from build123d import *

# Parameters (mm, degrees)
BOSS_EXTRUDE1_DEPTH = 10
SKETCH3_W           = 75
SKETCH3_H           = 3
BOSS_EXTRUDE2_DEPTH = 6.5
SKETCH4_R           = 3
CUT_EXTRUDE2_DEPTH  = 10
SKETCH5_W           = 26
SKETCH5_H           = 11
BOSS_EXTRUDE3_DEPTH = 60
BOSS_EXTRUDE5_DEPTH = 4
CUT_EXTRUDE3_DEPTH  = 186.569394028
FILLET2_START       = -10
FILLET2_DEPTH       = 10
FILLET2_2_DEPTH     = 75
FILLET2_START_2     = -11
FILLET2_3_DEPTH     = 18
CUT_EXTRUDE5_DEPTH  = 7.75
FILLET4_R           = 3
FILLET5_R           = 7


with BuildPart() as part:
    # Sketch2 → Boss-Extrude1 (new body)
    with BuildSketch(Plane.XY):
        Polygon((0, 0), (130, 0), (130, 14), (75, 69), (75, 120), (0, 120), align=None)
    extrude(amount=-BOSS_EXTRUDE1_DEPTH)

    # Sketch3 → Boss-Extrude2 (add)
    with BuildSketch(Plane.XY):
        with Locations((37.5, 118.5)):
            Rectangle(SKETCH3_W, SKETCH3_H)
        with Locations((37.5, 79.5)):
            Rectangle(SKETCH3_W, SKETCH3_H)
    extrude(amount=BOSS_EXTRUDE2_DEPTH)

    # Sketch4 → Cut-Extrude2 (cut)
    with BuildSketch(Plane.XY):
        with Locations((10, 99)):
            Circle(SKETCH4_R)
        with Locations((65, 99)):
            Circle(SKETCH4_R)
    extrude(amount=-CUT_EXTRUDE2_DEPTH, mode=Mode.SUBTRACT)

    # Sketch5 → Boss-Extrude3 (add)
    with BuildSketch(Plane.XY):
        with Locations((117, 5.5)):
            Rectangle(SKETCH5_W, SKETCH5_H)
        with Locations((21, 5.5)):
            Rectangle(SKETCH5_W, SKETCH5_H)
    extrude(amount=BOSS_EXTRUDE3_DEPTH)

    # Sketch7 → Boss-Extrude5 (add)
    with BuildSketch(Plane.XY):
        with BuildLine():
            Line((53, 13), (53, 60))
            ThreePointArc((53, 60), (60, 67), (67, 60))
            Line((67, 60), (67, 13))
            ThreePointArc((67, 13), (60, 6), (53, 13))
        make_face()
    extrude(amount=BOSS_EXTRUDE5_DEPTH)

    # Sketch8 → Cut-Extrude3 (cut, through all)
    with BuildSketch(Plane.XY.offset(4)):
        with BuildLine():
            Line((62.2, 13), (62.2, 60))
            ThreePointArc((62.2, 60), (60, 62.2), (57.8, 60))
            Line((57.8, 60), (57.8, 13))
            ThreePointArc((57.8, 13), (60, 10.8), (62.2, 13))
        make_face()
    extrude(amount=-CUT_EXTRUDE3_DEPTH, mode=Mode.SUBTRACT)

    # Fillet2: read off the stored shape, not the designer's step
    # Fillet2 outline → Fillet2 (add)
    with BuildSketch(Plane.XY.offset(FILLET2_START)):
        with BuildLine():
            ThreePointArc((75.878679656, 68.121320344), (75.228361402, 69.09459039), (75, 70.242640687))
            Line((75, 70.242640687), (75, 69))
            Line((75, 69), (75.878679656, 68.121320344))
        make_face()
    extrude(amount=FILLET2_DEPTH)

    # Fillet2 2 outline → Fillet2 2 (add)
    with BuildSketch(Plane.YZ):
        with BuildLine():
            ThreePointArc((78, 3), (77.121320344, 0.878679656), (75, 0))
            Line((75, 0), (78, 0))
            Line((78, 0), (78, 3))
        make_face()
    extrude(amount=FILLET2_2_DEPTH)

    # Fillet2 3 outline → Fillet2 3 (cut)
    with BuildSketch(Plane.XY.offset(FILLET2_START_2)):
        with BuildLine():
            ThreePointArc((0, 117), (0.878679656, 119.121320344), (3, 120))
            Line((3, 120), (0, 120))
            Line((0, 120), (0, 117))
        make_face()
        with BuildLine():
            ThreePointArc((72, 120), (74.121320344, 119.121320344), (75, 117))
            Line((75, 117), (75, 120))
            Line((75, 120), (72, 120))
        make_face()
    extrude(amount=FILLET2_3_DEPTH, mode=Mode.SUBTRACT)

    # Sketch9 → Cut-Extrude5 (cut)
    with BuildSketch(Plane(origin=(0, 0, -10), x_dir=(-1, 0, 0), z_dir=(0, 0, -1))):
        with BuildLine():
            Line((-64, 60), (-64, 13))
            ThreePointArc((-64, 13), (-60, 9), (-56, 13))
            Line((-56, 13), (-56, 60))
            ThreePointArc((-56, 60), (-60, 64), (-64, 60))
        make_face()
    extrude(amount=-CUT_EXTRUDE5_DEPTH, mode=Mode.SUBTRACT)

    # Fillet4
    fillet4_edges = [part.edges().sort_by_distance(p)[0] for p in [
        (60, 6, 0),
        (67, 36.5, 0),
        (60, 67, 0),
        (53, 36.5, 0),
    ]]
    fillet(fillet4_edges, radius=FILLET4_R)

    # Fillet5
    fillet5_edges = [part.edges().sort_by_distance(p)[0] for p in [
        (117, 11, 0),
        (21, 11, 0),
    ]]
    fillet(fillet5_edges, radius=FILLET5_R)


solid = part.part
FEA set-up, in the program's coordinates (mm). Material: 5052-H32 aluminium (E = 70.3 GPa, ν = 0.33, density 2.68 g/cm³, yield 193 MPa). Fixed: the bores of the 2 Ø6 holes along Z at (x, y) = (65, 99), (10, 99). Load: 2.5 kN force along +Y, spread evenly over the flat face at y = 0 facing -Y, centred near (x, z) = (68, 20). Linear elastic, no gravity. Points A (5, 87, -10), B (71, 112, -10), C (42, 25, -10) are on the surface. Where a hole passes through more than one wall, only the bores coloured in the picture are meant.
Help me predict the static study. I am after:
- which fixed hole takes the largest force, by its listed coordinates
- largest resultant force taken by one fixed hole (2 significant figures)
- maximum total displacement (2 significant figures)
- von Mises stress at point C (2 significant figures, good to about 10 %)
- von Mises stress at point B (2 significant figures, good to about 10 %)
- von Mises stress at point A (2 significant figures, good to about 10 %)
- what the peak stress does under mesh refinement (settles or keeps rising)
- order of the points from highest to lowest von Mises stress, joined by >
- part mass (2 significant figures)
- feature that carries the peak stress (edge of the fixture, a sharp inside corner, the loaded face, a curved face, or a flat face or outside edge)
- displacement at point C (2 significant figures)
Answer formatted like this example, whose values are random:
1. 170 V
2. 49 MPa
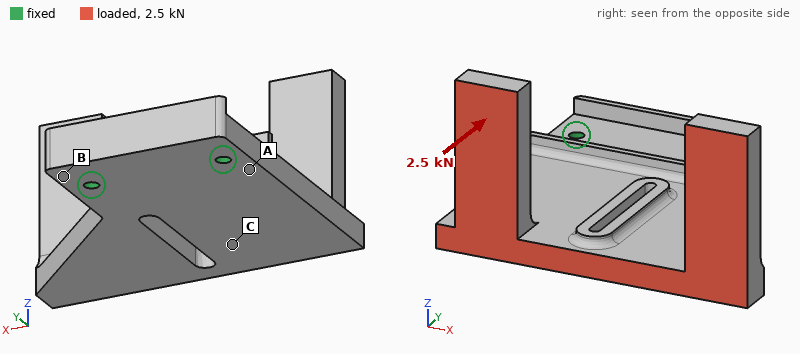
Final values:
1. (65, 99)
2. 2.6 kN
3. 1.3 mm
4. 28 MPa
5. 8.4 MPa
6. 53 MPa
7. keeps rising
8. A > C > B
9. 400 g
10. edge of the fixture
11. 0.40 mm
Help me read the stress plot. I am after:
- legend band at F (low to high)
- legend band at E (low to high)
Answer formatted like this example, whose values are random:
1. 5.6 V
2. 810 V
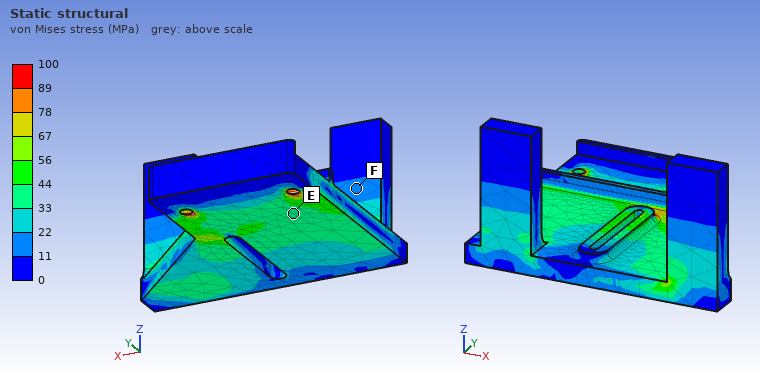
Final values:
1. 11 to 22 MPa
2. 33 to 44 MPa
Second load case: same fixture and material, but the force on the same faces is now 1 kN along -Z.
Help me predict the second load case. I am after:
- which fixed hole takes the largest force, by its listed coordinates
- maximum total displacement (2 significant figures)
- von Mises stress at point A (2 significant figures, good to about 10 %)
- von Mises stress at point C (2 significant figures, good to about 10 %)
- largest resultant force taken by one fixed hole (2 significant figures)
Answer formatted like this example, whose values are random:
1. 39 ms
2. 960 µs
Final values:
1. (65, 99)
2. 1.5 mm
3. 65 MPa
4. 20 MPa
5. 1.0 kN
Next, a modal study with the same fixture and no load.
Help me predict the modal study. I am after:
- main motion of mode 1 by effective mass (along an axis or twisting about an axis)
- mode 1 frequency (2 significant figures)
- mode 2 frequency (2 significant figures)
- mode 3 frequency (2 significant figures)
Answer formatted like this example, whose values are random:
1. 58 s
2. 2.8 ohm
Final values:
1. along Z
2. 380 Hz
3. 640 Hz
4. 1200 Hz
